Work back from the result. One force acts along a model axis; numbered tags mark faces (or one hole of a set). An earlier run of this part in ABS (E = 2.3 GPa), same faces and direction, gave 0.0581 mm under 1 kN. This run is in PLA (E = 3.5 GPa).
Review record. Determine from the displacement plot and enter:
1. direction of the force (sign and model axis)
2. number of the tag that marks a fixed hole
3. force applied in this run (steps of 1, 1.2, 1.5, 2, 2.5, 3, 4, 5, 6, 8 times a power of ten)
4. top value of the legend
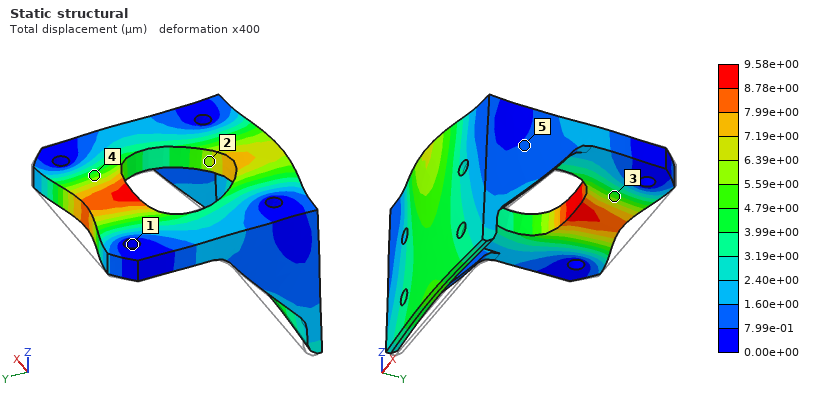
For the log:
-Y
1
250 N
9.58e+00 µm
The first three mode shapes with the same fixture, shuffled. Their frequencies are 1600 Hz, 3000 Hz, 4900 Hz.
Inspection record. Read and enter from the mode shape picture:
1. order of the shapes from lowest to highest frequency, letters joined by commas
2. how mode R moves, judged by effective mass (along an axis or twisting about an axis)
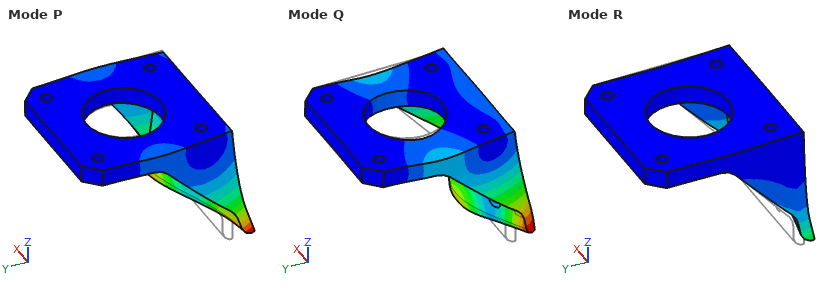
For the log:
R, P, Q
along Y
